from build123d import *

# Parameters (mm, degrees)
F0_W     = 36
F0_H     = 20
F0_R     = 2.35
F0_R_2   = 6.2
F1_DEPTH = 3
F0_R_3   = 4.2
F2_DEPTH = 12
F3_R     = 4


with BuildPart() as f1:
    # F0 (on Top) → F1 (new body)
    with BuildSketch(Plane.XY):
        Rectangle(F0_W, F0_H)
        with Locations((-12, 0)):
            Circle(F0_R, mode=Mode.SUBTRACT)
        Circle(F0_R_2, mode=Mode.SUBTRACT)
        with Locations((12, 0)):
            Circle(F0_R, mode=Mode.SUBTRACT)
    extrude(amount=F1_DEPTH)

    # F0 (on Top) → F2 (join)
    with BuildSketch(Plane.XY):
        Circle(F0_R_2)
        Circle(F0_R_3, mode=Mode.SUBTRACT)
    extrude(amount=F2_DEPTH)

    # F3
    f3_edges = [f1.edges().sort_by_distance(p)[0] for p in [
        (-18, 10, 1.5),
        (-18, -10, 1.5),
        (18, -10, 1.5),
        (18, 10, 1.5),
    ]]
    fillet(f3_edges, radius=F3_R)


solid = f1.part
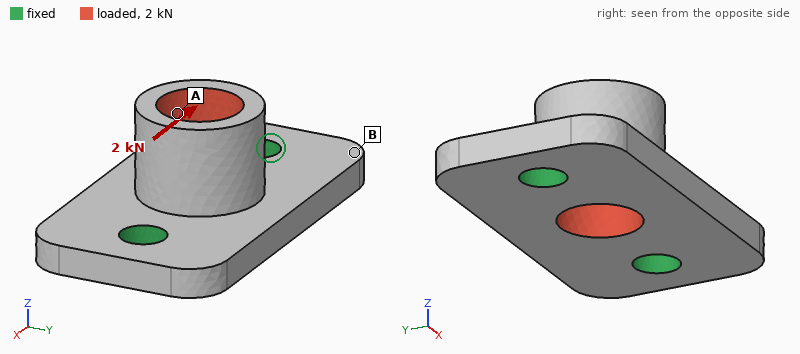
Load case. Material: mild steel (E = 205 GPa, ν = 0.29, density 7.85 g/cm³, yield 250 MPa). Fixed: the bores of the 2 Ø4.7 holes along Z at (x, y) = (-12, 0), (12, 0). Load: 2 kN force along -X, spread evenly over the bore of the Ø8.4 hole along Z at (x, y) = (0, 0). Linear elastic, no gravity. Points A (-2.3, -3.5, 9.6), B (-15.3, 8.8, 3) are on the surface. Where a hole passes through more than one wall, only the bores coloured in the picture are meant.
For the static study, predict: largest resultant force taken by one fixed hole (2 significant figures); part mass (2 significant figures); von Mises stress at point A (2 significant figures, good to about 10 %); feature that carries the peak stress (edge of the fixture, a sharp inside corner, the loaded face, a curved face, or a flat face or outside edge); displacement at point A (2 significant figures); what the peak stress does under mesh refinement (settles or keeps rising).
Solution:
1.1 kN
19 g
30 MPa
edge of the fixture
6.8 µm
keeps rising
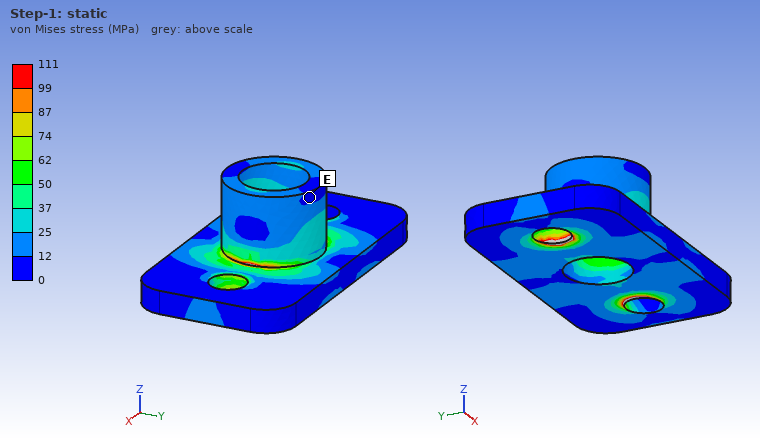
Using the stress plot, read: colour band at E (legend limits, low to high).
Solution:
0 to 12 MPa
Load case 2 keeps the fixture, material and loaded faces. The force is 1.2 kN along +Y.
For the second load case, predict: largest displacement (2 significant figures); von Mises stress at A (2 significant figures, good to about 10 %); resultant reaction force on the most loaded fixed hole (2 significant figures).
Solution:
18 µm
13 MPa
600 N
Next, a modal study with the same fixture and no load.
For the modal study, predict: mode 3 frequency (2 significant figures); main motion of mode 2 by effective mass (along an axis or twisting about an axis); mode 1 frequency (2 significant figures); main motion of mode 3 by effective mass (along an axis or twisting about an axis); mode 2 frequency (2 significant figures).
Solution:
32 kHz
along Z
15 kHz
along X
24 kHz
